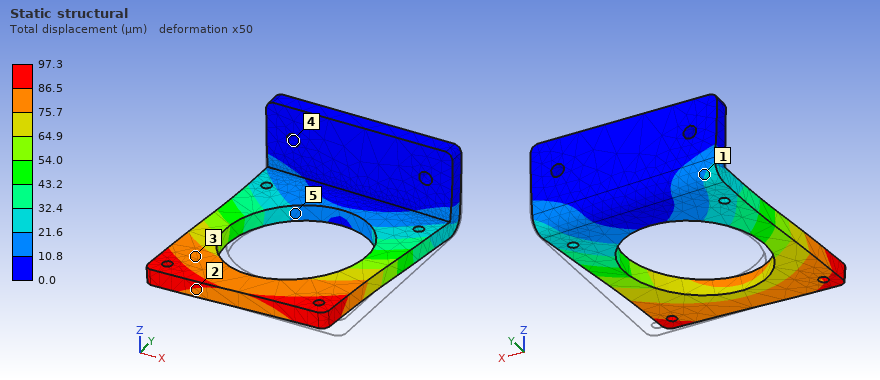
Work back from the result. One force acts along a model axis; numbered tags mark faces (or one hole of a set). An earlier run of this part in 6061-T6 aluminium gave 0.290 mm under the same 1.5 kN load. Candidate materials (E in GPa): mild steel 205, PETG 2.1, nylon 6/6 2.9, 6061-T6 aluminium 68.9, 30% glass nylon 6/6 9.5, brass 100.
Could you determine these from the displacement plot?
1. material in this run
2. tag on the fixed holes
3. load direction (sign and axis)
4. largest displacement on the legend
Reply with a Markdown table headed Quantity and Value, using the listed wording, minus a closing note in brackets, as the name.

| Quantity | Value |
|---|---|
| material in this run | mild steel |
| tag on the fixed holes | 4 |
| load direction | -X |
| largest displacement on the legend | 97.3 µm |
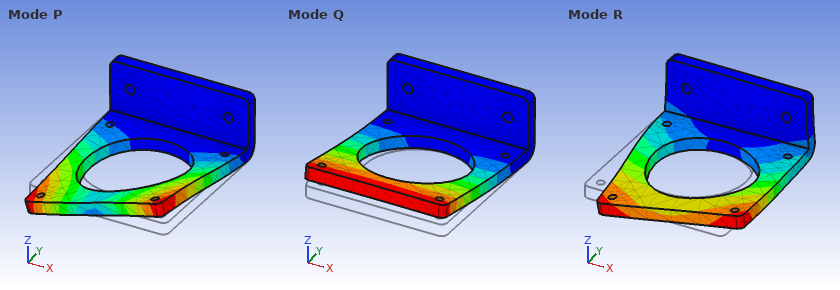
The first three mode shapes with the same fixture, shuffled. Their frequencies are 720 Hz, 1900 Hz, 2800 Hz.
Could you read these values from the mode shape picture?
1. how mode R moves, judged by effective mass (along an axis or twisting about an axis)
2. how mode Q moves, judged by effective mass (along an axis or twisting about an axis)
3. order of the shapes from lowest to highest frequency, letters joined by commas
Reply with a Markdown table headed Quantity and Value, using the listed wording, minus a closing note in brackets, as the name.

| Quantity | Value |
|---|---|
| how mode R moves, judged by effective mass | along X |
| how mode Q moves, judged by effective mass | along Z |
| order of the shapes from lowest to highest frequency, letters joined by commas | Q, P, R |
